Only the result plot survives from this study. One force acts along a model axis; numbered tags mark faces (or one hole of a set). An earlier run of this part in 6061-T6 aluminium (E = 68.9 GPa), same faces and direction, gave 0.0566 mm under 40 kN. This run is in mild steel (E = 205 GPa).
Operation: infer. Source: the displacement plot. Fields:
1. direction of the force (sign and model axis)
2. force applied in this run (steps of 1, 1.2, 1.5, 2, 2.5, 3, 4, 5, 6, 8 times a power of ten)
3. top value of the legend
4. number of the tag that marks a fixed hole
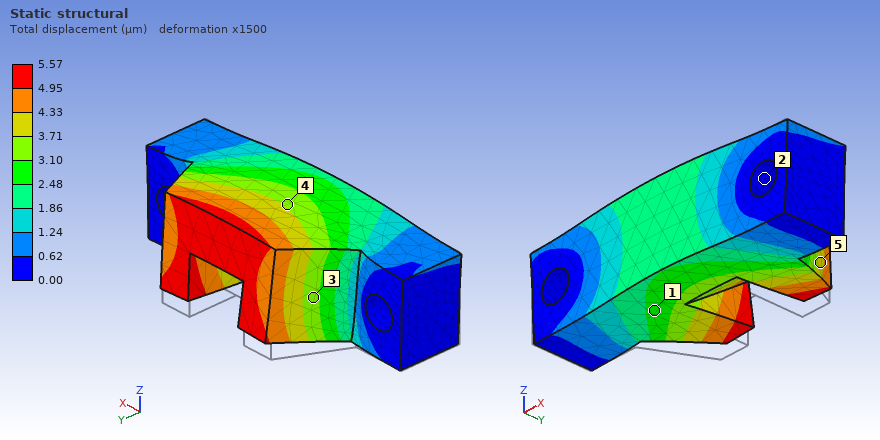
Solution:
+Z
12 kN
5.57 µm
2
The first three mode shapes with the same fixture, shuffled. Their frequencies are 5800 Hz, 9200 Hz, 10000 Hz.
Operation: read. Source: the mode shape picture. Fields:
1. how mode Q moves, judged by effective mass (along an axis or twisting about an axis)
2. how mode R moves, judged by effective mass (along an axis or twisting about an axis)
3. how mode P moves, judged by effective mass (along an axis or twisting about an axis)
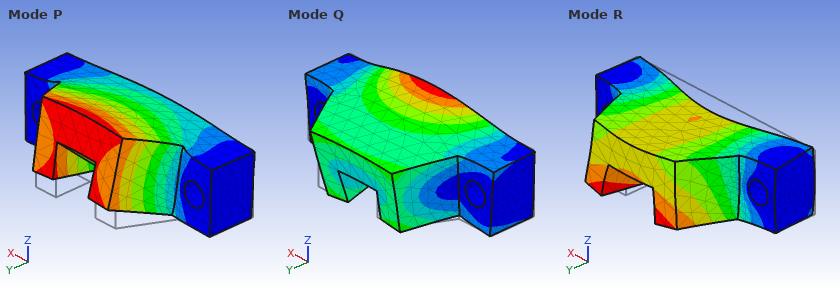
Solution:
along Z
along Y
along Z
